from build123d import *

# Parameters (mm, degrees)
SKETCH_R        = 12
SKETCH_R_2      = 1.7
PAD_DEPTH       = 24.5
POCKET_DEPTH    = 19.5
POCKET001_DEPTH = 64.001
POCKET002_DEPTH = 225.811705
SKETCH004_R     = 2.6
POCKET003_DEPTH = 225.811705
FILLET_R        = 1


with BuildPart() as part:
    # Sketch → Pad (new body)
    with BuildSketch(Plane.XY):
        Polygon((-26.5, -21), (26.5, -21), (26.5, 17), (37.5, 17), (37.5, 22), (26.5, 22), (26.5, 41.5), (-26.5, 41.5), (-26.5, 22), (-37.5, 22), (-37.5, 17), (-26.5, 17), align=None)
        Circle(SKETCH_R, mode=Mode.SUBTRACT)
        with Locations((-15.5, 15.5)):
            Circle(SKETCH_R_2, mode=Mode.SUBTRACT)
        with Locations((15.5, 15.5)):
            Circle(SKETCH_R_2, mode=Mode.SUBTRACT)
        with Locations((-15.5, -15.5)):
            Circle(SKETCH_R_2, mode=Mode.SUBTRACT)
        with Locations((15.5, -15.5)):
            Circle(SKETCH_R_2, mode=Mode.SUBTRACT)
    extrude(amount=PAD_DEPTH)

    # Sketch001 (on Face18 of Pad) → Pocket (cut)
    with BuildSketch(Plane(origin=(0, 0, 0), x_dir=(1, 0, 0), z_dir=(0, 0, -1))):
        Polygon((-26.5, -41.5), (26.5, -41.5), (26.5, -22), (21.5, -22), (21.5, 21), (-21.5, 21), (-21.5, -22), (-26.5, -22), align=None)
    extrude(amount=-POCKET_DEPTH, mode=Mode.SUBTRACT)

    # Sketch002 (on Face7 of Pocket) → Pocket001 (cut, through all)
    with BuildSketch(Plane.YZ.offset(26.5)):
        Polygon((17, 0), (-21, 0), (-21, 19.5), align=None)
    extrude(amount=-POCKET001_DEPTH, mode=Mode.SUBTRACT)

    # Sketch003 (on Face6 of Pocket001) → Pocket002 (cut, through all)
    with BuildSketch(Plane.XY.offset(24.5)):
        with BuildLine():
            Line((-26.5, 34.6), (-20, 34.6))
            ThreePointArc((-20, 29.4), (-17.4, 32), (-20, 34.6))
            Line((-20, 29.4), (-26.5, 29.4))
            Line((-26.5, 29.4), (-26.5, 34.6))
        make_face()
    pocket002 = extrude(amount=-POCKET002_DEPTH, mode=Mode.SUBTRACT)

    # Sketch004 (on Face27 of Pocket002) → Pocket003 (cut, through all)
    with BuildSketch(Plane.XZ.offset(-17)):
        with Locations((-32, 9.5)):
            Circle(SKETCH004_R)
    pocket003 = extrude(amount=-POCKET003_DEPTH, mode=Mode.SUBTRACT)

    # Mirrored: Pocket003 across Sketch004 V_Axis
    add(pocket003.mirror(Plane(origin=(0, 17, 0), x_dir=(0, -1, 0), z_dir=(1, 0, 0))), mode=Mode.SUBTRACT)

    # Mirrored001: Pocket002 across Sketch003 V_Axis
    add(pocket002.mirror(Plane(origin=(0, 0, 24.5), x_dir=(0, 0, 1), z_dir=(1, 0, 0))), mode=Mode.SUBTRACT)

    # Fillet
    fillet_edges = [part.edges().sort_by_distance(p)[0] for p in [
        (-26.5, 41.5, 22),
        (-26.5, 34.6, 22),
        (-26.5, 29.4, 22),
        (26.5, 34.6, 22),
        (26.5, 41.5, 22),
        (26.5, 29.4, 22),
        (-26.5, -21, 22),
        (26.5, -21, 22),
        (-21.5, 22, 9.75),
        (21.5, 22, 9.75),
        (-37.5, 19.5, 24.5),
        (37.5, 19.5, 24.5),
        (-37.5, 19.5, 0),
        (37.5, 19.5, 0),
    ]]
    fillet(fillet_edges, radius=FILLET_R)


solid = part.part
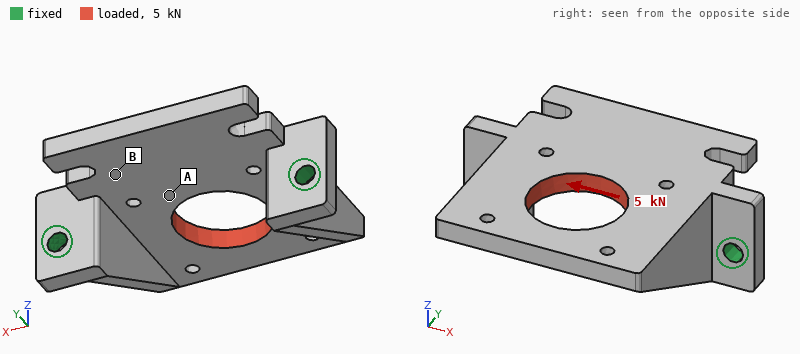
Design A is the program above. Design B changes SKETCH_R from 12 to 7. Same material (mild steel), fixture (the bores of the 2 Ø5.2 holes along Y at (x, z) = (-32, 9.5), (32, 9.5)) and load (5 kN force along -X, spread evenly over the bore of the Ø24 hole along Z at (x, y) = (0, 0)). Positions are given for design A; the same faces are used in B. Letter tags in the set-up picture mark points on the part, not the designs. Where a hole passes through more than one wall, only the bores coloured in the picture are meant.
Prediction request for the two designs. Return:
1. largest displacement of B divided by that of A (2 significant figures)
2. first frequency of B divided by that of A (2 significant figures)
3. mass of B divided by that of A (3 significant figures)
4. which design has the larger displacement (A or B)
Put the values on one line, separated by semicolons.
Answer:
0.87; 0.96; 1.07; A
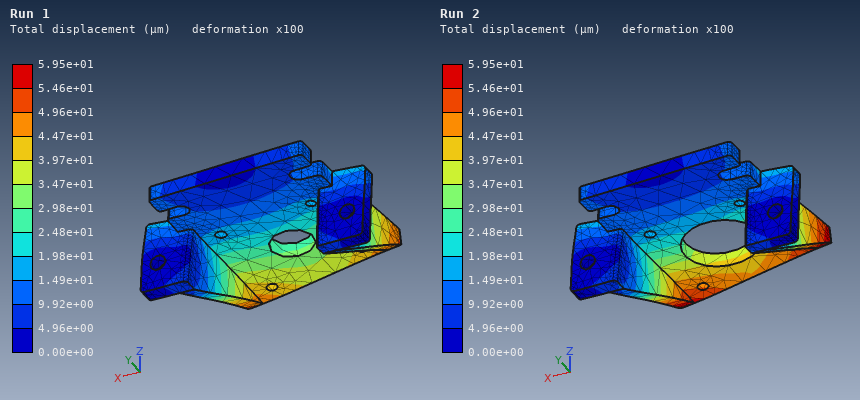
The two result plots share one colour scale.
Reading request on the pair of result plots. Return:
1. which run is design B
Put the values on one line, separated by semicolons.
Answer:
Run 1
